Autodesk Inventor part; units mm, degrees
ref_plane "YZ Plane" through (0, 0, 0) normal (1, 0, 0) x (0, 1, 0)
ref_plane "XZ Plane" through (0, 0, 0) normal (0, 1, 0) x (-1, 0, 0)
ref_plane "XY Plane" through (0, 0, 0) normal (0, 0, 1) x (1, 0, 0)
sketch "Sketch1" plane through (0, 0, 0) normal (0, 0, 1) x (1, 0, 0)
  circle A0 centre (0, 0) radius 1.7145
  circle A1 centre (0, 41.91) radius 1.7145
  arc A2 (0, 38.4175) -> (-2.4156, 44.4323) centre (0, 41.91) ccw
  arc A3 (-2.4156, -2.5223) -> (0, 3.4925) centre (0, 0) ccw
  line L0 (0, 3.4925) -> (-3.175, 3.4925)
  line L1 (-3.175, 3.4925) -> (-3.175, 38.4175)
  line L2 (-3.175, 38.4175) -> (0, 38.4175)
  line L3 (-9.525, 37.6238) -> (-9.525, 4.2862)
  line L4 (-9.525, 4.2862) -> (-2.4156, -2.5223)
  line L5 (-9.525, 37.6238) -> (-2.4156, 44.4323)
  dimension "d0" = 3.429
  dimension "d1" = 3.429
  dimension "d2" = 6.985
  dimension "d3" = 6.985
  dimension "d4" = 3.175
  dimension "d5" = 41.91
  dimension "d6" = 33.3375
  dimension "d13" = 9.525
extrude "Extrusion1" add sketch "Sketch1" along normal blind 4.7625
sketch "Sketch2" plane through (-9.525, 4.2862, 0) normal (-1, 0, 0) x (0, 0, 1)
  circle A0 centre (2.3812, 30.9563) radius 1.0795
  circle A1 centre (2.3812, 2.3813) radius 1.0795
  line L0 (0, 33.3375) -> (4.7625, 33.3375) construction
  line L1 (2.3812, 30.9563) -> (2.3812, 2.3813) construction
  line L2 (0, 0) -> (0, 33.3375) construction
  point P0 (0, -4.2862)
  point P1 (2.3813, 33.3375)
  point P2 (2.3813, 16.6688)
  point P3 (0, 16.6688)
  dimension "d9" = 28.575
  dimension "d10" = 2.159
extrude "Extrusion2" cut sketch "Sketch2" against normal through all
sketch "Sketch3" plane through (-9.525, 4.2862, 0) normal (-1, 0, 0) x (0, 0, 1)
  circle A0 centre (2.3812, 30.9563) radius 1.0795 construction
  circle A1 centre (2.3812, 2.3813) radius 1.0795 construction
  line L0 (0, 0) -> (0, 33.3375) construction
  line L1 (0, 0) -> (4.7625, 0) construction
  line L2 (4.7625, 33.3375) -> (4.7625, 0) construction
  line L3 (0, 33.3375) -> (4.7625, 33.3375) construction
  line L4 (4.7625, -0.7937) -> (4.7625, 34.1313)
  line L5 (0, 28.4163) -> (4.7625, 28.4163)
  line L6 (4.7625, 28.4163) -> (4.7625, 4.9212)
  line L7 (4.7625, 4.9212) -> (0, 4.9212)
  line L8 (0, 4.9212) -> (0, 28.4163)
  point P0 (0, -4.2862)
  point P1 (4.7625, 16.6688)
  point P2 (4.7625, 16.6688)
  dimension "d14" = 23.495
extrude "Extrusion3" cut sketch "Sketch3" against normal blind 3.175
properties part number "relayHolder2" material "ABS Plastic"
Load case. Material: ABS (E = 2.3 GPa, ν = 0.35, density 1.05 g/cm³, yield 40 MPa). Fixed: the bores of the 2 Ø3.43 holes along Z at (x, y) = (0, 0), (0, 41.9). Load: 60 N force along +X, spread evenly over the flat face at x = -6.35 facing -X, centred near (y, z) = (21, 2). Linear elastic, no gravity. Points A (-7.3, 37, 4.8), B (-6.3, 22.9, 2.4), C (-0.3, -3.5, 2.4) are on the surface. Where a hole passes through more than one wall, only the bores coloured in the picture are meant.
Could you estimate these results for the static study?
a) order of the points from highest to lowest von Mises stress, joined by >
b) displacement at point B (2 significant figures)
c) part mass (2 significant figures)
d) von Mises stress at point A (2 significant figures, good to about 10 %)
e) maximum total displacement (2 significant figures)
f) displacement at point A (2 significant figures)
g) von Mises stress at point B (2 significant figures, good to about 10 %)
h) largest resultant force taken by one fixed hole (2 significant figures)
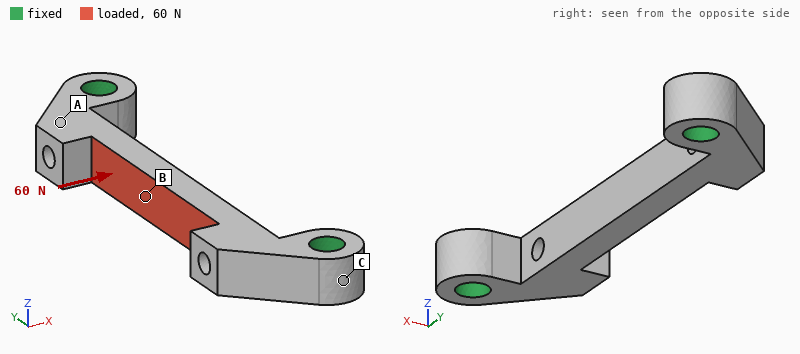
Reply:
B > A > C
0.40 mm
1.1 g
5.9 MPa
0.42 mm
0.087 mm
17 MPa
38 N
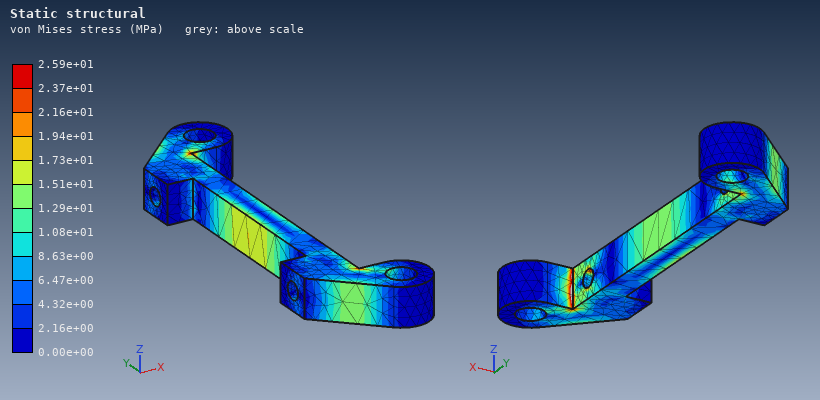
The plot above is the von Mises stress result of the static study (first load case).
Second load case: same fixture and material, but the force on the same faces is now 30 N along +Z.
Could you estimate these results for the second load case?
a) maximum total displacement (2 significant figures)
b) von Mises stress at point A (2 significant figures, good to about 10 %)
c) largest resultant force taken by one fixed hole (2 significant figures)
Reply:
0.18 mm
3.0 MPa
15 N
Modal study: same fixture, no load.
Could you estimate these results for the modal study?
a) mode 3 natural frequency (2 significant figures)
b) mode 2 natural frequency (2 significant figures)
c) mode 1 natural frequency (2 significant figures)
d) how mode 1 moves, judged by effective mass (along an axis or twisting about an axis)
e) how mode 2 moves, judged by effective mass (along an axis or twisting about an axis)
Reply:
6700 Hz
3500 Hz
3300 Hz
along X
along Z
